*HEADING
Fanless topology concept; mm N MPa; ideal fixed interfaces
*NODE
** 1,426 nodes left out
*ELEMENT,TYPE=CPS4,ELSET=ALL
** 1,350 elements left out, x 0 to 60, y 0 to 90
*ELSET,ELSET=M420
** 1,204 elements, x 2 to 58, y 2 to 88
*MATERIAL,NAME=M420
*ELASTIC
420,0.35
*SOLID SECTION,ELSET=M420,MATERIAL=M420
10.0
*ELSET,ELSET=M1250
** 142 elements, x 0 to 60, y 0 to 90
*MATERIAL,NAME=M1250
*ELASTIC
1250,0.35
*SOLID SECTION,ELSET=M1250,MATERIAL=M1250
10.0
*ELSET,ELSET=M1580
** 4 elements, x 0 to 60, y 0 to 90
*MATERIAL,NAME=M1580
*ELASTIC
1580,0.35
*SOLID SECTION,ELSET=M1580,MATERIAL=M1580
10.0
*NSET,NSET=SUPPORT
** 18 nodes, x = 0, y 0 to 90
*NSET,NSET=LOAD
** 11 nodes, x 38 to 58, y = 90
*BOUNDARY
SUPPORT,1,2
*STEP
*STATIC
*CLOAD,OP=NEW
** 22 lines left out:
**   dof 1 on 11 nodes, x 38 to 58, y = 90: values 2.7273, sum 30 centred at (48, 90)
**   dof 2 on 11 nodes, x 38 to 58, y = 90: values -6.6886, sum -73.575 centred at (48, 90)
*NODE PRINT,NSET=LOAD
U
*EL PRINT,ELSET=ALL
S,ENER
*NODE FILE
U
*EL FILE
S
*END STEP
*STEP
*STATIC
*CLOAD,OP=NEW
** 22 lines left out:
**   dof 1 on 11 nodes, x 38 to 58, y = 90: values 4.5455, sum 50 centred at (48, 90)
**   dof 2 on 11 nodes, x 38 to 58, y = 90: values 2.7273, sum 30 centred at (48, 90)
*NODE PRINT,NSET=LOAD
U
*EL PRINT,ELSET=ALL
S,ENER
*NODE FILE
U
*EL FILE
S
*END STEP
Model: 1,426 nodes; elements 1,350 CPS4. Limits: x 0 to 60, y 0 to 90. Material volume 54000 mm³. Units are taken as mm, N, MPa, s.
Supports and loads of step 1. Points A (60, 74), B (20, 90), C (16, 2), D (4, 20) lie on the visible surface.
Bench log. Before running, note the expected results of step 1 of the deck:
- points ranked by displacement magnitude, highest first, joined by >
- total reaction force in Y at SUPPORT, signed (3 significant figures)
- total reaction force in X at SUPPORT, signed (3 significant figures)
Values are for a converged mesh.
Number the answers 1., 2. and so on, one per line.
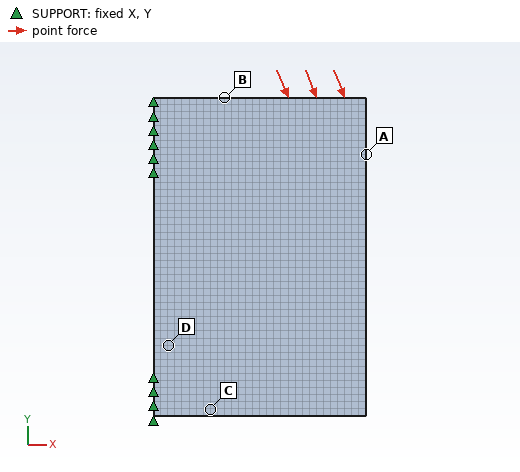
1. A > B > C > D
2. 73.6 N
3. -30.0 N
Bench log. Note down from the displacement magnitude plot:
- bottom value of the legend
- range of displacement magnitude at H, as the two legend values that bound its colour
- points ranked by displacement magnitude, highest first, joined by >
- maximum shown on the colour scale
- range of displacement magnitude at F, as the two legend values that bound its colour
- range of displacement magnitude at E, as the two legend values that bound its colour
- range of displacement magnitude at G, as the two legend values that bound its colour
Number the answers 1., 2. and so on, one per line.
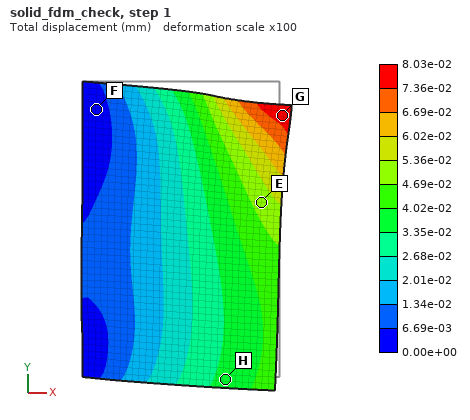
1. 0.00e+00 mm
2. 3.35e-02 to 4.02e-02 mm
3. G > E > H > F
4. 8.03e-02 mm
5. 0.00e+00 to 6.69e-03 mm
6. 4.69e-02 to 5.36e-02 mm
7. 7.36e-02 to 8.03e-02 mm
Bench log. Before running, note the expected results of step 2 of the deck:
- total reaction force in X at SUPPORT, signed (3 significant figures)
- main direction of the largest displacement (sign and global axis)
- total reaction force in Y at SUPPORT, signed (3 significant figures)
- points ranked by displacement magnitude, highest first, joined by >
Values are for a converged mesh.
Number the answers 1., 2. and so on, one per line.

1. -50.0 N
2. +X
3. -30.0 N
4. A > B > C > D
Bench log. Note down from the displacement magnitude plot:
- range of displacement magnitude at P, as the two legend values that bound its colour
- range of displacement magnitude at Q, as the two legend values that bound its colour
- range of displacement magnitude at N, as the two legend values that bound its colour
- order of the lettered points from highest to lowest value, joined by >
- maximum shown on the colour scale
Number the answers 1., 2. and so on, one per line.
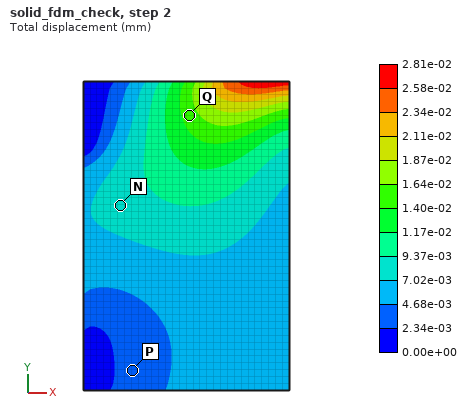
1. 2.34e-03 to 4.68e-03 mm
2. 1.40e-02 to 1.64e-02 mm
3. 7.02e-03 to 9.37e-03 mm
4. Q > N > P
5. 2.81e-02 mm
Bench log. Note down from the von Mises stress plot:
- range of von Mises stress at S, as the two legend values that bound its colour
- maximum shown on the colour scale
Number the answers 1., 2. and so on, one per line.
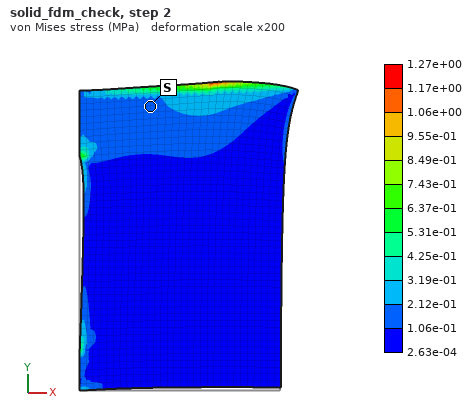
1. 1.06e-01 to 2.12e-01 MPa
2. 1.27e+00 MPa
